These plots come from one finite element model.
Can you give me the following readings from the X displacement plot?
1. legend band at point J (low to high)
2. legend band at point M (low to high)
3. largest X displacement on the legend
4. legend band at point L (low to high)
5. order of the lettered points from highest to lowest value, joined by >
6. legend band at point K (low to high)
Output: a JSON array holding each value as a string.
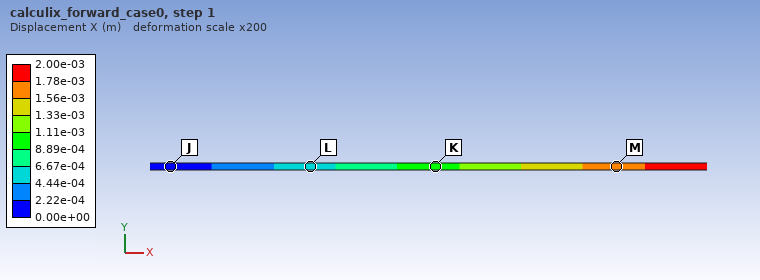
["0.00e+00 to 2.22e-04 m", "1.56e-03 to 1.78e-03 m", "2.00e-03 m", "4.44e-04 to 6.67e-04 m", "M > K > L > J", "8.89e-04 to 1.11e-03 m"]
